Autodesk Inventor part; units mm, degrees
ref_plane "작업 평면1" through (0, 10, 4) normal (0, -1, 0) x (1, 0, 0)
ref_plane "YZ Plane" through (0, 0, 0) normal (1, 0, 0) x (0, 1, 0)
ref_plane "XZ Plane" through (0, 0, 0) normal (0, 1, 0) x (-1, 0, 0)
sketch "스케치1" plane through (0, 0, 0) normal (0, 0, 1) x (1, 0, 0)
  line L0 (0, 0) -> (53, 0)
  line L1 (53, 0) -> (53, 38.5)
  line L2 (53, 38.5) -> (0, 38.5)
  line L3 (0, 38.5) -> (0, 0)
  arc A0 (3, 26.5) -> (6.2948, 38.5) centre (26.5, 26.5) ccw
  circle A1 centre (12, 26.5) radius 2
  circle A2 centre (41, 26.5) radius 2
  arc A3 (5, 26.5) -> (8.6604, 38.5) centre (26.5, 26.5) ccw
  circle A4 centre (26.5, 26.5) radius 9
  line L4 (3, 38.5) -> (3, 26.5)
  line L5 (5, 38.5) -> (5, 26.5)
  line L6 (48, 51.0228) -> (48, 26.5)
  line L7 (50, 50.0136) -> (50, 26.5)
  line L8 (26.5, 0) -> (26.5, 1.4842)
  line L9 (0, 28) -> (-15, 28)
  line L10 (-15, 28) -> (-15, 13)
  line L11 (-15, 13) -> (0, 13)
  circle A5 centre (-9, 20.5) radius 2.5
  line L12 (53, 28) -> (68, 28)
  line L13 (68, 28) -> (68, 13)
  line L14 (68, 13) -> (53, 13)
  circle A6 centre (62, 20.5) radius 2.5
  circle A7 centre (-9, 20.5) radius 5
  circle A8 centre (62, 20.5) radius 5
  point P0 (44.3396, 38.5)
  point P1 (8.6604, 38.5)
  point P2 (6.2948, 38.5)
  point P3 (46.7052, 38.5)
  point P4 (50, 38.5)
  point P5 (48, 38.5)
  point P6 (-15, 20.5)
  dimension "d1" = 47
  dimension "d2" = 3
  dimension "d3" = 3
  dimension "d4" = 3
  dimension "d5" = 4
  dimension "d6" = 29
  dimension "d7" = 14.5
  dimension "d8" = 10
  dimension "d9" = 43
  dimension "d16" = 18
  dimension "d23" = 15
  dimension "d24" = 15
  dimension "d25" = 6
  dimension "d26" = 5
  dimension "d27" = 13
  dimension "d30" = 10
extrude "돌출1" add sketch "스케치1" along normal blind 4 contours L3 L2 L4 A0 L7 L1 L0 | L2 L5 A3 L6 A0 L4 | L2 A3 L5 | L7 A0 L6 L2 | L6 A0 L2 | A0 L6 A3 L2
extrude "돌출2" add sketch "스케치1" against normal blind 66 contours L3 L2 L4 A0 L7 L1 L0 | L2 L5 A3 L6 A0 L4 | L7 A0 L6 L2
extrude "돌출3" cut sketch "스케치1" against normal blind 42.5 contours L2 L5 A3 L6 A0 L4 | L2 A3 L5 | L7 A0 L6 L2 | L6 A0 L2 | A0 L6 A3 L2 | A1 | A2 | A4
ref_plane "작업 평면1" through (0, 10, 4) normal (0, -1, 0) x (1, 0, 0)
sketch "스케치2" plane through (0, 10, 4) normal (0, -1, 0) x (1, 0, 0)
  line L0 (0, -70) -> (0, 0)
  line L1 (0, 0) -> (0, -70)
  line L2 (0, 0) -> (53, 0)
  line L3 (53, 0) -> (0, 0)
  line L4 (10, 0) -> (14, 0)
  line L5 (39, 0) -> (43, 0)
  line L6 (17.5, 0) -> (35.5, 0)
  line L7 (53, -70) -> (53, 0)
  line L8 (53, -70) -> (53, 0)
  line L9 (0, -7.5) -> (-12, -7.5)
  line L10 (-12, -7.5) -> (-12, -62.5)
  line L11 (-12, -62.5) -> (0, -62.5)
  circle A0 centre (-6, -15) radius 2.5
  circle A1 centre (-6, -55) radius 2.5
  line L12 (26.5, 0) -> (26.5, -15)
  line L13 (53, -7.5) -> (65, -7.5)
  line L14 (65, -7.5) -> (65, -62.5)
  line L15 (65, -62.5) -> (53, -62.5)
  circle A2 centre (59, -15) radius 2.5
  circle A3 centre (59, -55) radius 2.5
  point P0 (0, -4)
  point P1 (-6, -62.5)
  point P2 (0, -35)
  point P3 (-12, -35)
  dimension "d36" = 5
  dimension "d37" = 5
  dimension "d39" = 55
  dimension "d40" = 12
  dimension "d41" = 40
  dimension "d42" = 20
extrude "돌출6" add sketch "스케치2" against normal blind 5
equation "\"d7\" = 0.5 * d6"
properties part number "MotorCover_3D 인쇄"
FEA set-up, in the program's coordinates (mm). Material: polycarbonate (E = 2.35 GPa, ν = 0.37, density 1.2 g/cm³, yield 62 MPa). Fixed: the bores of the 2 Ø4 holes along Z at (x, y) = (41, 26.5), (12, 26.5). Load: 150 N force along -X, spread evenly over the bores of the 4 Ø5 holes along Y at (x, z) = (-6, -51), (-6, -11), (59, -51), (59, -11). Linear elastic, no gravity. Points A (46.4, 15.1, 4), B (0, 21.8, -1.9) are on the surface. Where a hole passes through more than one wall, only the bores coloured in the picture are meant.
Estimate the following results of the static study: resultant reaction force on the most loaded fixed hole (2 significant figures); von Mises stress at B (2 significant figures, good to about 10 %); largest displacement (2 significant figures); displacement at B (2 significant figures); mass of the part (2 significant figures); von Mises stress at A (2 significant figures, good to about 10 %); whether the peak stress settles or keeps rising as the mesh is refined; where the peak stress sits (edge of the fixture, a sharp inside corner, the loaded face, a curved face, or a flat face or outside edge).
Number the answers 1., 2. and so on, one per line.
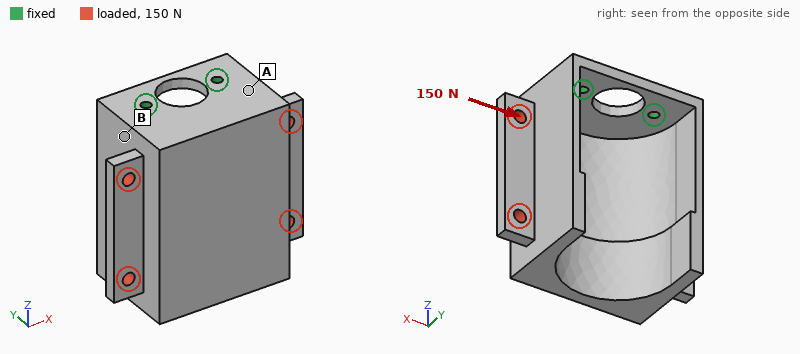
1. 150 N
2. 1.4 MPa
3. 1.1 mm
4. 0.20 mm
5. 69 g
6. 2.9 MPa
7. keeps rising
8. edge of the fixture
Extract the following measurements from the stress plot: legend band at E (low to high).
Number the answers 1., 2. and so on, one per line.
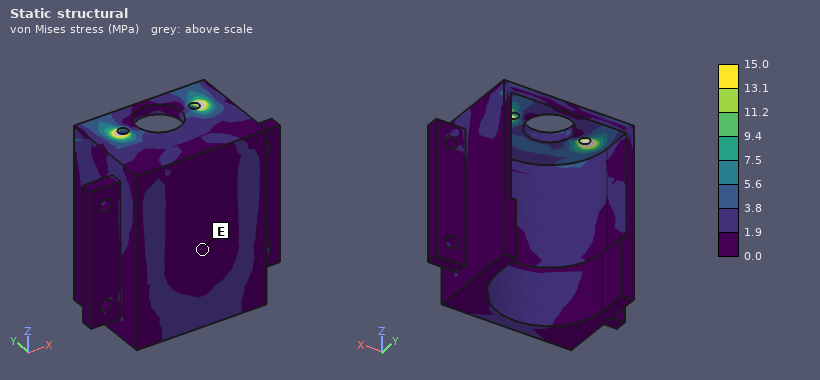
1. 0.0 to 1.9 MPa
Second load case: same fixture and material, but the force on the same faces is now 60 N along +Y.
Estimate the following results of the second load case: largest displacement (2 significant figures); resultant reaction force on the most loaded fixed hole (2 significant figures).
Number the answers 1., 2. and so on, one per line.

1. 1.2 mm
2. 31 N
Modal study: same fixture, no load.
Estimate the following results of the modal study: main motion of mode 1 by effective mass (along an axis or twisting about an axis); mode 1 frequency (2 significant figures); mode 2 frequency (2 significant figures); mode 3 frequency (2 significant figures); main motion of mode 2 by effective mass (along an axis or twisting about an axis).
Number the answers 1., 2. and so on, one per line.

1. along Y
2. 150 Hz
3. 280 Hz
4. 750 Hz
5. along X
